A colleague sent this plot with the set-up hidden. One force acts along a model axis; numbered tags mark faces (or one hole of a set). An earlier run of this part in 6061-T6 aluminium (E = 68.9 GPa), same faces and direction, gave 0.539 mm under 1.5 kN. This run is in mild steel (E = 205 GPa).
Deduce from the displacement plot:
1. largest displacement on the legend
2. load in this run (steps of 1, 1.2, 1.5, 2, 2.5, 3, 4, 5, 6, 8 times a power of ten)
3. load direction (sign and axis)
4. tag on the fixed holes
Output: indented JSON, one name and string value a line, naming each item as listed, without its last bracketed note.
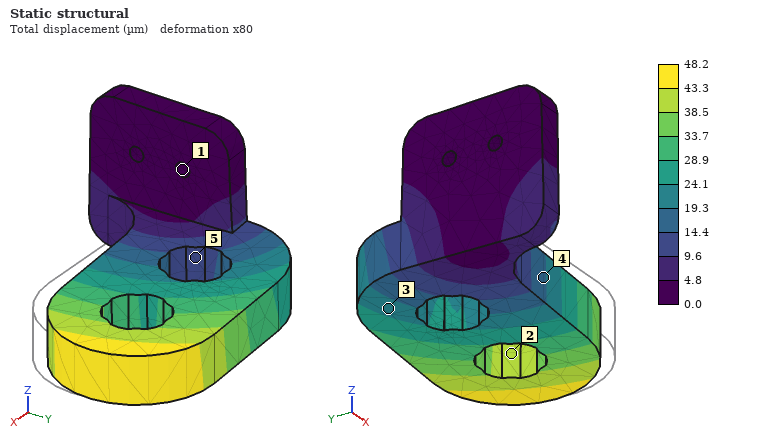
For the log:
{
  "largest displacement on the legend": "48.2 µm",
  "load in this run": "400 N",
  "load direction": "+Y",
  "tag on the fixed holes": "1"
}
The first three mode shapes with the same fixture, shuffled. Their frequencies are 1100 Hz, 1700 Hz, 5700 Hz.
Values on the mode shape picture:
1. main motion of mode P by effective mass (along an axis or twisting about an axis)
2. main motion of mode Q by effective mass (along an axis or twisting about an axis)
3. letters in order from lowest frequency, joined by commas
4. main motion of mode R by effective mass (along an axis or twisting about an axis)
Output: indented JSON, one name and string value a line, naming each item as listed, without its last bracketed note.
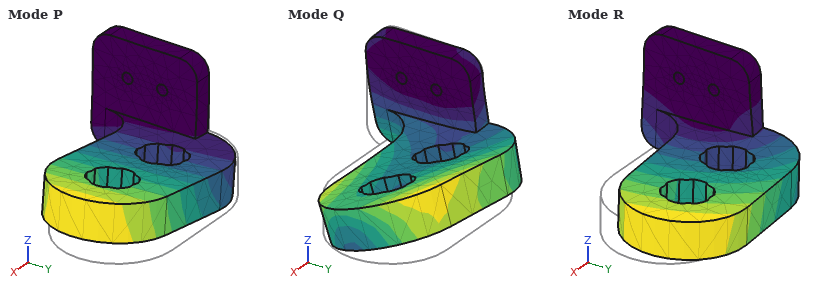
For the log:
{
  "main motion of mode P by effective mass": "along Z",
  "main motion of mode Q by effective mass": "along X",
  "letters in order from lowest frequency, joined by commas": "P, R, Q",
  "main motion of mode R by effective mass": "along Y"
}
